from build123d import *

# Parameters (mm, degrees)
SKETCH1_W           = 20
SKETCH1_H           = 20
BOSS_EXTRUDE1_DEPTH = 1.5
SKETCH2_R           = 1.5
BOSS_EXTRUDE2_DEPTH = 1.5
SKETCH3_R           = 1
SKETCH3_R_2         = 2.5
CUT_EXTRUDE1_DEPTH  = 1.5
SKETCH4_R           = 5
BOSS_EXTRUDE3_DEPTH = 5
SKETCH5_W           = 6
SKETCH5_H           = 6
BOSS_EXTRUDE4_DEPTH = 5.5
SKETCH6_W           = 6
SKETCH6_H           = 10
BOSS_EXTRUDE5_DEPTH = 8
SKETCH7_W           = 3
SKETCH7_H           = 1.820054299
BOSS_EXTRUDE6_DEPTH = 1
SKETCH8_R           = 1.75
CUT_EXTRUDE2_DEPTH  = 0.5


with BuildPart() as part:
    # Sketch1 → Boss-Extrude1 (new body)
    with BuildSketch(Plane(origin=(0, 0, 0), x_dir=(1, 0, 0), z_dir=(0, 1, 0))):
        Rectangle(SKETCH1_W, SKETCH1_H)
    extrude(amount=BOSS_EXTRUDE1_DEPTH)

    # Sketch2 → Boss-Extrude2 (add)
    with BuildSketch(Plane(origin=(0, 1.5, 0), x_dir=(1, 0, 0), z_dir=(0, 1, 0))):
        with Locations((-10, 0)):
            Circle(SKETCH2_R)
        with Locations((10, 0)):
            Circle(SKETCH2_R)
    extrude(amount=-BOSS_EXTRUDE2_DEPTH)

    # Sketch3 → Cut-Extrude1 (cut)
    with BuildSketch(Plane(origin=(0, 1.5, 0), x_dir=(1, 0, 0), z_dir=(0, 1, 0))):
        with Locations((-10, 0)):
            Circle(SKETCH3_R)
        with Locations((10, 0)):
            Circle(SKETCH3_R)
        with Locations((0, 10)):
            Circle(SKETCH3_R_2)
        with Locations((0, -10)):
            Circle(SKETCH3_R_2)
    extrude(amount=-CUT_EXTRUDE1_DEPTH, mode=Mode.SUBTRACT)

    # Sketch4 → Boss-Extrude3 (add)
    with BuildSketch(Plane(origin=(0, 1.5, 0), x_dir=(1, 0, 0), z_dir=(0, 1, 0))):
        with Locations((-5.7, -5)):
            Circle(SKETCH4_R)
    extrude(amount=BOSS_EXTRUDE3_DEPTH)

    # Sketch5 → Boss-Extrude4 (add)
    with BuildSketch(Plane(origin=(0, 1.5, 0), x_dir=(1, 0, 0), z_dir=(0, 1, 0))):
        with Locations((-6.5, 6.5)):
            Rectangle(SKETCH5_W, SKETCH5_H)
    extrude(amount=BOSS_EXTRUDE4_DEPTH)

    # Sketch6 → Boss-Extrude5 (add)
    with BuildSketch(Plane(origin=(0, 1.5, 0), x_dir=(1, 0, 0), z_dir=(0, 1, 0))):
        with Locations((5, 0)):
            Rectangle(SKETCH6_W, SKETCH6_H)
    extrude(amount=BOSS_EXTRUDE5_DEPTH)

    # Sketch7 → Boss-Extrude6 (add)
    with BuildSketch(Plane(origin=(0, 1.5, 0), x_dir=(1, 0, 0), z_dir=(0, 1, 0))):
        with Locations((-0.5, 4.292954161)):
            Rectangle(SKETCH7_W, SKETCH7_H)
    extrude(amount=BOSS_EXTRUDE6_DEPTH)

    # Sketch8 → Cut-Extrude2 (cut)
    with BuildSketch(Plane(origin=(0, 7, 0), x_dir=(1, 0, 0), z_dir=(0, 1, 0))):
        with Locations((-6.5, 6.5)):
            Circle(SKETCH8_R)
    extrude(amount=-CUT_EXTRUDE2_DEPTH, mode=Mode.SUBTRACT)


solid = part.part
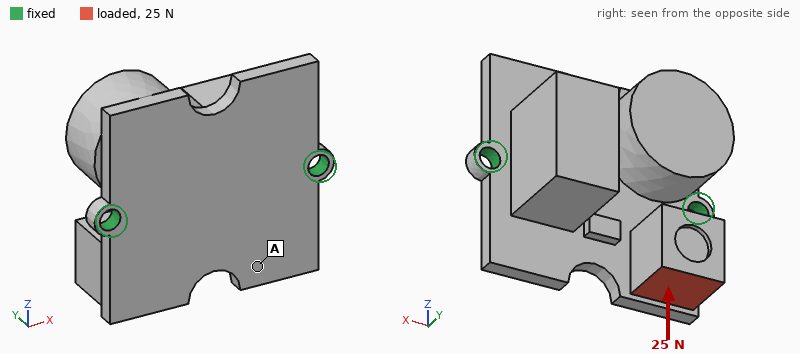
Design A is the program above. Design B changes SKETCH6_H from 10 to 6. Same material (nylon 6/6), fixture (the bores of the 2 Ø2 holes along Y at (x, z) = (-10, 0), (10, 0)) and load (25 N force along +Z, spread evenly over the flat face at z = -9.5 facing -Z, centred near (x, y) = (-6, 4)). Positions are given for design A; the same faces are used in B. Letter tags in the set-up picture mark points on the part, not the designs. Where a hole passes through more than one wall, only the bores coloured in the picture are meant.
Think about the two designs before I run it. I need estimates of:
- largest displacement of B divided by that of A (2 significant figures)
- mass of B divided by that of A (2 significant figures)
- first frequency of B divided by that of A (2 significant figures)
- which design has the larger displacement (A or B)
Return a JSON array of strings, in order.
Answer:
["1.1", "0.88", "1.0", "B"]
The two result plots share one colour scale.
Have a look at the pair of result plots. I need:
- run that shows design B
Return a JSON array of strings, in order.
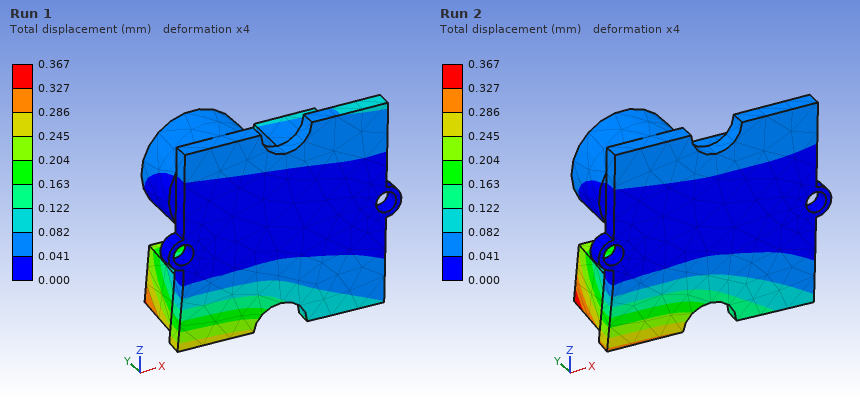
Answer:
["Run 2"]
